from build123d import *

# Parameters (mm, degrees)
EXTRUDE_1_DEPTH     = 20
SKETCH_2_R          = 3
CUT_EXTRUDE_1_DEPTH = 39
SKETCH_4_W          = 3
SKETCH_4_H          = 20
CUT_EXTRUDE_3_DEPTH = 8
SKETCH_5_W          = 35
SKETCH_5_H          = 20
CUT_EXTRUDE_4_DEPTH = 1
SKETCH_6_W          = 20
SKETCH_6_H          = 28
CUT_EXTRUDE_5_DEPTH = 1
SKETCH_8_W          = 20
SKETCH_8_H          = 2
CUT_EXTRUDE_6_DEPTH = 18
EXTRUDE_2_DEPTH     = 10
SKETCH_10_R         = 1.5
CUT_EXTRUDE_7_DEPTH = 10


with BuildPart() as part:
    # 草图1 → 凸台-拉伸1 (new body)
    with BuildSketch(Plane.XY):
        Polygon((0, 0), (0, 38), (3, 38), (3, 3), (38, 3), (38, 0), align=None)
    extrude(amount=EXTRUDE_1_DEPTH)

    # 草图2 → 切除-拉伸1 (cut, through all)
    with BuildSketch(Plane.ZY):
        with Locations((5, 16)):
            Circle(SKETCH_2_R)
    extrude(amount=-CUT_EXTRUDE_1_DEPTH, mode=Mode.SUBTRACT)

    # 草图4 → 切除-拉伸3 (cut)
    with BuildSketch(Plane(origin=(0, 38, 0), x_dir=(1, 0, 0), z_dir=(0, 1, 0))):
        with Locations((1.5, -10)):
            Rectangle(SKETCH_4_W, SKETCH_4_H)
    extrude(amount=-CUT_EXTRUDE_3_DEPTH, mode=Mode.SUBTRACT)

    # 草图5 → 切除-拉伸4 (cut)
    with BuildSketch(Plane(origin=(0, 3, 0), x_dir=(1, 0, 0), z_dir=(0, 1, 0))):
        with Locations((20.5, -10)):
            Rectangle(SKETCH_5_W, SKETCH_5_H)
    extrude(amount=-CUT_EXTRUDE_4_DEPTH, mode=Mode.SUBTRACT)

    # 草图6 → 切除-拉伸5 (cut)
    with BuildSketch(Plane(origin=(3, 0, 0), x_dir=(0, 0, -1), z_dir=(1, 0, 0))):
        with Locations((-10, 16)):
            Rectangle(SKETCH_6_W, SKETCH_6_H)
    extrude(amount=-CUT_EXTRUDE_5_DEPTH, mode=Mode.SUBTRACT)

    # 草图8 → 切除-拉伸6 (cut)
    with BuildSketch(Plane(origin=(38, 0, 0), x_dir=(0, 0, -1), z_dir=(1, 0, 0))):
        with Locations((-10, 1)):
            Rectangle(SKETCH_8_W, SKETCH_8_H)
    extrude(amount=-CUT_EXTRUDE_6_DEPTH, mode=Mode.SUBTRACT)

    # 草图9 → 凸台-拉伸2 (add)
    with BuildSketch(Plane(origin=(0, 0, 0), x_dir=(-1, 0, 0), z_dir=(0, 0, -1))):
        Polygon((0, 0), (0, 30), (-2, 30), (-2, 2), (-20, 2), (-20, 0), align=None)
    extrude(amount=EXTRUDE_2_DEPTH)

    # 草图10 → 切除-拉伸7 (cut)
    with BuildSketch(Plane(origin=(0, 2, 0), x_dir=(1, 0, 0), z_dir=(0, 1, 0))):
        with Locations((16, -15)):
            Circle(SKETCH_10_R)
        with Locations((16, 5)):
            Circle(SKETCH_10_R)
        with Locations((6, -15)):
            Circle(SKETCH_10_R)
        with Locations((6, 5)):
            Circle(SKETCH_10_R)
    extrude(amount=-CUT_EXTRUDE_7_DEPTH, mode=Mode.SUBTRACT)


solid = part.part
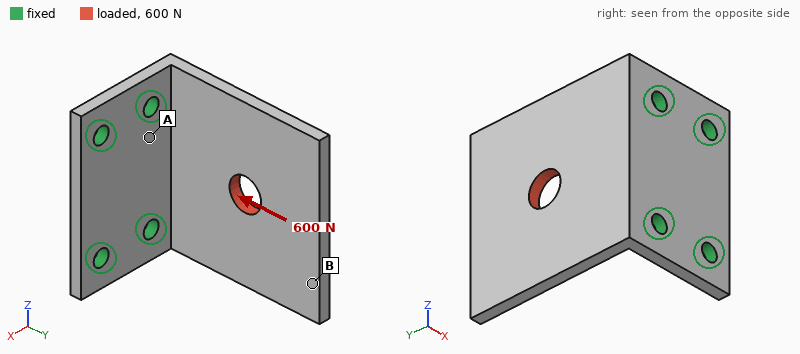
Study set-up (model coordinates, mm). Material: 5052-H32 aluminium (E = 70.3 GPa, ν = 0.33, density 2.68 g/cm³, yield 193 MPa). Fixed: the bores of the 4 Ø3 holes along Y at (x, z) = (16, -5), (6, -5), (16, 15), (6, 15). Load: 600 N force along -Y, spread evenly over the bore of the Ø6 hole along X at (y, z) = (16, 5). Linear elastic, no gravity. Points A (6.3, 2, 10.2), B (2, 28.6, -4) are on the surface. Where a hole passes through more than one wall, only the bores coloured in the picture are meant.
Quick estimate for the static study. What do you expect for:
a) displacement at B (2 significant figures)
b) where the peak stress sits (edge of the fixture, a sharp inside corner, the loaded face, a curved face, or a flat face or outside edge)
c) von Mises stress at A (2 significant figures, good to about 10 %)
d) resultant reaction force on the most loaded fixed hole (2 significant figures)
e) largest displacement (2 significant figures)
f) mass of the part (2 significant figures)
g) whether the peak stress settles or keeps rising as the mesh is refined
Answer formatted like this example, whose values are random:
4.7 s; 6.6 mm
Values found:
0.13 mm; edge of the fixture; 43 MPa; 330 N; 0.14 mm; 7.4 g; keeps rising
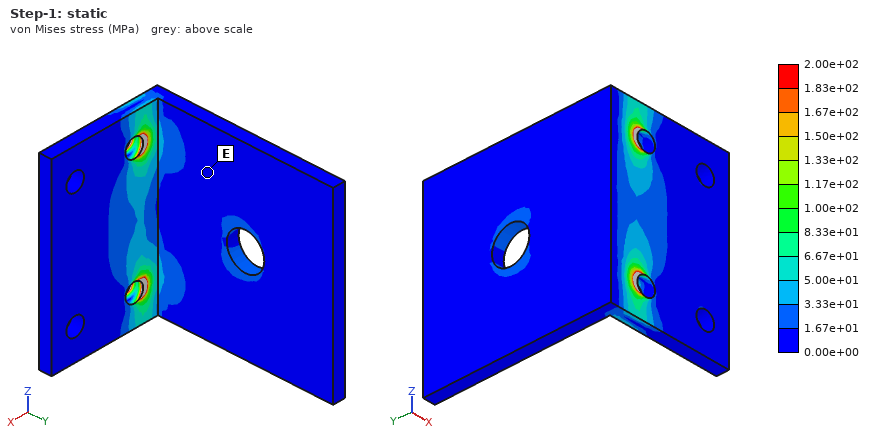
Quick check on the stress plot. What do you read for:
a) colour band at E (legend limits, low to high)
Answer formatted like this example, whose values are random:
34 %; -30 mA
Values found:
0.00e+00 to 1.67e+01 MPa
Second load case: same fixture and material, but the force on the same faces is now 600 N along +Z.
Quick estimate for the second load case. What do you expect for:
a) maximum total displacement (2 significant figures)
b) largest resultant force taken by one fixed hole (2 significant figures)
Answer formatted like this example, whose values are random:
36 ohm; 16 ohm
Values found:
95 µm; 540 N
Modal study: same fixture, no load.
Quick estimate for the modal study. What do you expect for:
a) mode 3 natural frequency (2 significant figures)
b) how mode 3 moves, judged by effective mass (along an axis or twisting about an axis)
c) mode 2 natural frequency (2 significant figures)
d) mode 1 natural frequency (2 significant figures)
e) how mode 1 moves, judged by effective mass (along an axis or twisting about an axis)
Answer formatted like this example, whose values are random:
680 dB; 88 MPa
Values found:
8100 Hz; along Z; 4100 Hz; 1600 Hz; along X
